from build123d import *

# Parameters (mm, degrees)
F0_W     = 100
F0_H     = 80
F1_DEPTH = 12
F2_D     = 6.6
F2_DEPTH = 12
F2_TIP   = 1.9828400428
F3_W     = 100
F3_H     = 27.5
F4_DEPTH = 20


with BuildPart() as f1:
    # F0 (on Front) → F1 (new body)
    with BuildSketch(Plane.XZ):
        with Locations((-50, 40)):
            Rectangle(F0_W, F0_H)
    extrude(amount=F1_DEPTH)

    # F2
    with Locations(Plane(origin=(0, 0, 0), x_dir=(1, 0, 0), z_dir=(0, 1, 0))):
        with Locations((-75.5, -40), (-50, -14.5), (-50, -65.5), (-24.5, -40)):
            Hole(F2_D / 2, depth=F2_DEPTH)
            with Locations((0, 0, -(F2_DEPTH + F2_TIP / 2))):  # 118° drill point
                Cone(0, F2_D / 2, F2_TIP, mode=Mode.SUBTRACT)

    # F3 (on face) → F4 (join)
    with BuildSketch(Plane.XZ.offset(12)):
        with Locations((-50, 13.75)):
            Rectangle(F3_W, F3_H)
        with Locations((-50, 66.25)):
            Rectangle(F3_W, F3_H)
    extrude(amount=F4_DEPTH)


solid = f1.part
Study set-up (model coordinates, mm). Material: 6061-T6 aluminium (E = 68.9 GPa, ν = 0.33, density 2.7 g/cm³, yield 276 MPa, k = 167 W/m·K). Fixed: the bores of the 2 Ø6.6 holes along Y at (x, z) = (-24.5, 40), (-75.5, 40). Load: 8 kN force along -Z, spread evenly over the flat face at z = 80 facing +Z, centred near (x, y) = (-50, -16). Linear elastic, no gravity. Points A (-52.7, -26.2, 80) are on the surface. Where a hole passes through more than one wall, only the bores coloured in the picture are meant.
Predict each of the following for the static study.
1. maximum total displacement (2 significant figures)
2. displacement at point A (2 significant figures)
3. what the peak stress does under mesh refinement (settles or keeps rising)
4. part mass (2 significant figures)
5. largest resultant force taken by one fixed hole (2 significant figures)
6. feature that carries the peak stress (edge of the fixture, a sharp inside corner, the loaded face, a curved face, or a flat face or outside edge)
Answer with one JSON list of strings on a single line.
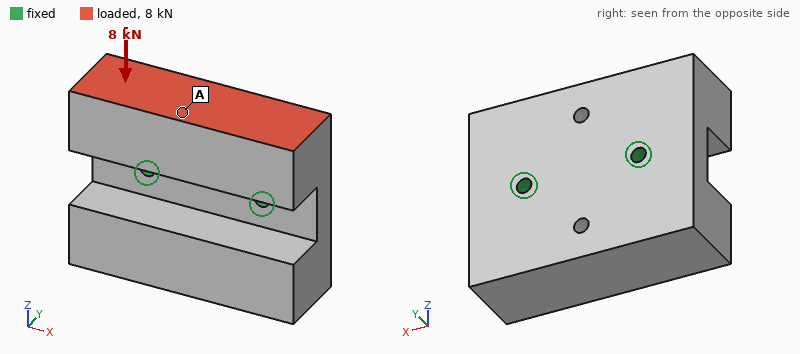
["77 µm", "71 µm", "keeps rising", "550 g", "4.0 kN", "edge of the fixture"]
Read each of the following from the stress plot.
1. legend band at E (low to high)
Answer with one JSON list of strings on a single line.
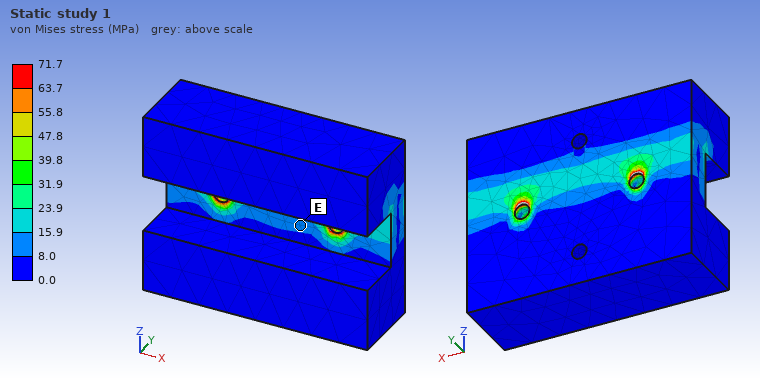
["8.0 to 15.9 MPa"]
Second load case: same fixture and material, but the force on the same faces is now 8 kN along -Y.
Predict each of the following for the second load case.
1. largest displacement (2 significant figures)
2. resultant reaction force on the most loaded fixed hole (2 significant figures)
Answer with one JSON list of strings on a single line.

["0.26 mm", "4.0 kN"]
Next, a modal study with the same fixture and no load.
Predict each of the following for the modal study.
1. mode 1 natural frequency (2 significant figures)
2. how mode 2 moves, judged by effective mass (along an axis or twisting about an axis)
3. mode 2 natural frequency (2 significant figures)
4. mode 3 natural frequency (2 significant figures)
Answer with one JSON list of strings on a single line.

["2300 Hz", "along Y", "3300 Hz", "5400 Hz"]
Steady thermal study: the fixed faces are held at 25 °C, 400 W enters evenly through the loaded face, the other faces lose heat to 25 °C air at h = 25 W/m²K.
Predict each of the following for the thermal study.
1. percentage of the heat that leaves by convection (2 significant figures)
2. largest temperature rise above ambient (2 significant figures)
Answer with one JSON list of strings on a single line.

["5.0 %", "68 K"]
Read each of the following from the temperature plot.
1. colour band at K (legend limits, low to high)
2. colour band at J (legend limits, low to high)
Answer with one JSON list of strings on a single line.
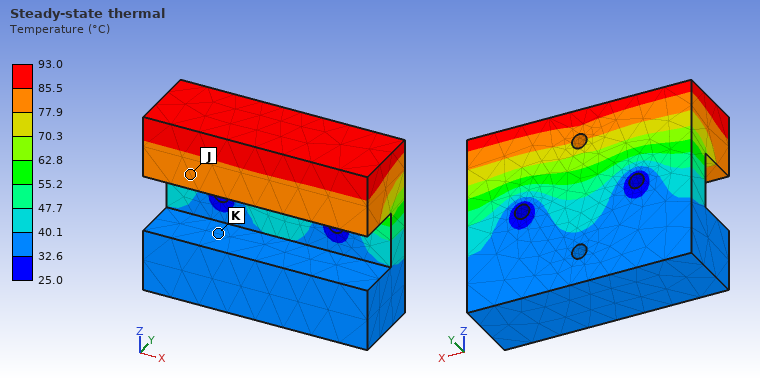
["32.6 to 40.1 °C", "77.9 to 85.5 °C"]
